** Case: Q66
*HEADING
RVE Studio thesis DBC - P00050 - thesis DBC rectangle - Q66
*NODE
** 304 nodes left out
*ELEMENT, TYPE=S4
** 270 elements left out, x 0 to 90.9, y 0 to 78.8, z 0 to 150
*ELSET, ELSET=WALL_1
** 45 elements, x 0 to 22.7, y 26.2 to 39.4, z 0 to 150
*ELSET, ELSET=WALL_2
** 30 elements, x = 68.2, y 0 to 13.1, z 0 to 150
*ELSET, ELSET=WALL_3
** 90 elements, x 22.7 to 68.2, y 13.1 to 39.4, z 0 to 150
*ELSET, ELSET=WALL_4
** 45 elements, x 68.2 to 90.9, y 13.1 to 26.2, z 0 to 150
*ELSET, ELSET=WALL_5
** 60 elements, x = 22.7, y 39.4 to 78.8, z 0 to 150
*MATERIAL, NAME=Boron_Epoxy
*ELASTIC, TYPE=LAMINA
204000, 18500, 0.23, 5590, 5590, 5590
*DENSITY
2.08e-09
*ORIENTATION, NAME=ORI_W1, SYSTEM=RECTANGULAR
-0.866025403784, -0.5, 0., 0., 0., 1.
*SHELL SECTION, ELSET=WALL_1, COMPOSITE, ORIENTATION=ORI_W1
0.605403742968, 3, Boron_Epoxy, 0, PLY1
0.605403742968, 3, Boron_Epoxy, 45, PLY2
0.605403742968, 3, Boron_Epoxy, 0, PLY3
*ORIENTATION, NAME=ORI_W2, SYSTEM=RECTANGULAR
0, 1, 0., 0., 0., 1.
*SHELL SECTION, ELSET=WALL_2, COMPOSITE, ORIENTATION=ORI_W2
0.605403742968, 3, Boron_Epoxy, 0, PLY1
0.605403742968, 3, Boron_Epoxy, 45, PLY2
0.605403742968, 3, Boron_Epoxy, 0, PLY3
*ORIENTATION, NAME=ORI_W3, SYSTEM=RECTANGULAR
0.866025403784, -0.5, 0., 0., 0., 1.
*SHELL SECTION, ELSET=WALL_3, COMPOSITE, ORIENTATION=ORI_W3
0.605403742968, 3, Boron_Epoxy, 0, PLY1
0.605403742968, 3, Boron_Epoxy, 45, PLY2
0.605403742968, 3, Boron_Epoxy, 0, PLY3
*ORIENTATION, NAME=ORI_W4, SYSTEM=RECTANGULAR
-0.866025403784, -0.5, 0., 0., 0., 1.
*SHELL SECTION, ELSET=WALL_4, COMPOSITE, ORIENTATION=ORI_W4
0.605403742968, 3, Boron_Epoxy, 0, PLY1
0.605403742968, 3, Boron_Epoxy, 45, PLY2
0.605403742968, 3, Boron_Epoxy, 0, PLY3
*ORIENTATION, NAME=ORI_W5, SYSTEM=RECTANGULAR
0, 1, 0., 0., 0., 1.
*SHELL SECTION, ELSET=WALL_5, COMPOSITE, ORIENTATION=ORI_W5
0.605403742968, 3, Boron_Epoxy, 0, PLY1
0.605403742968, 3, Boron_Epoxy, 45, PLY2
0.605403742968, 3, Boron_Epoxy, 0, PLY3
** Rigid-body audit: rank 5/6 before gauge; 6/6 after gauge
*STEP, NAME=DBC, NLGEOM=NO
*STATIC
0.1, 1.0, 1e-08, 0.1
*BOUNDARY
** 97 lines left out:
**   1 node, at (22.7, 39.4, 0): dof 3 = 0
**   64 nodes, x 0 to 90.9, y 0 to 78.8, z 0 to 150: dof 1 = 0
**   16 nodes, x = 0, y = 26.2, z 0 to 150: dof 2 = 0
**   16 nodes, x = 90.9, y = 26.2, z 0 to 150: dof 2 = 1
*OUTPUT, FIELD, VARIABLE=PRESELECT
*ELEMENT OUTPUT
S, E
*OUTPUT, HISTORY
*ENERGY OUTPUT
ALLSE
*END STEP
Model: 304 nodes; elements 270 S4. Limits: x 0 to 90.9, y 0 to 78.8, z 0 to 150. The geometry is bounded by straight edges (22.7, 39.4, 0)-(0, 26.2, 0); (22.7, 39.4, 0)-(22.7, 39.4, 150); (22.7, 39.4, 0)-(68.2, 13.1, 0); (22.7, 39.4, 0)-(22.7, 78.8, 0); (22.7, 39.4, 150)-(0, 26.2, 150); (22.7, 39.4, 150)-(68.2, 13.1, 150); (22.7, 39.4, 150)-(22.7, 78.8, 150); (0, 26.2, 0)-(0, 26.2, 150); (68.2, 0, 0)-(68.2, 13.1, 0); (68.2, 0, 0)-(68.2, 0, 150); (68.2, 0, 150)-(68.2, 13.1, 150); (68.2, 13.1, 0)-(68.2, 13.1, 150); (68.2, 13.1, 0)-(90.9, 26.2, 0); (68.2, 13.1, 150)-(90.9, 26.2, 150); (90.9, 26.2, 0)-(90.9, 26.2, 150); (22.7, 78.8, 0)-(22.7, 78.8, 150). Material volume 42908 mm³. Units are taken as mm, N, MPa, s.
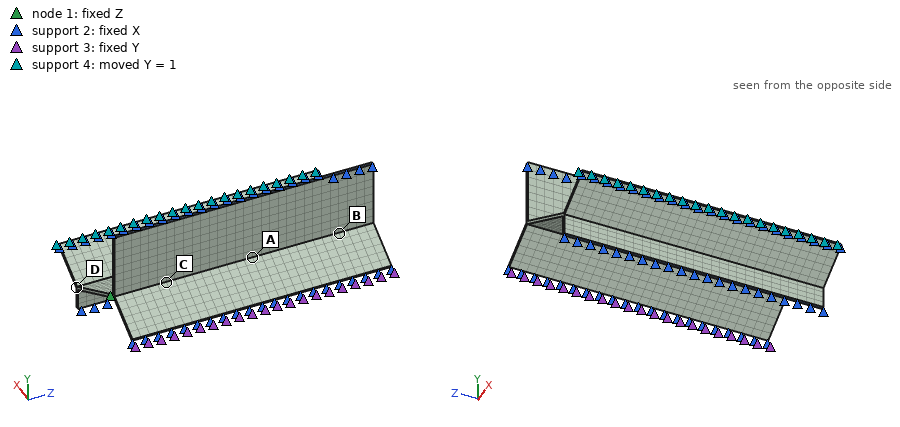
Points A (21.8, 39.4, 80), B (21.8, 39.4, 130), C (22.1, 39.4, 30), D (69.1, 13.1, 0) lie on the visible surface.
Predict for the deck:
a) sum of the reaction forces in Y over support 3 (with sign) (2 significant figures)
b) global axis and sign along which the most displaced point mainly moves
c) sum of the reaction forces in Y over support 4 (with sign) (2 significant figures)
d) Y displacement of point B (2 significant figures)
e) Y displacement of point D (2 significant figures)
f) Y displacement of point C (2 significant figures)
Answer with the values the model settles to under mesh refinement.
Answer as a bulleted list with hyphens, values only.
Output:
- -600 N
- +Y
- 600 N
- 0.40 mm
- 0.92 mm
- 0.41 mm
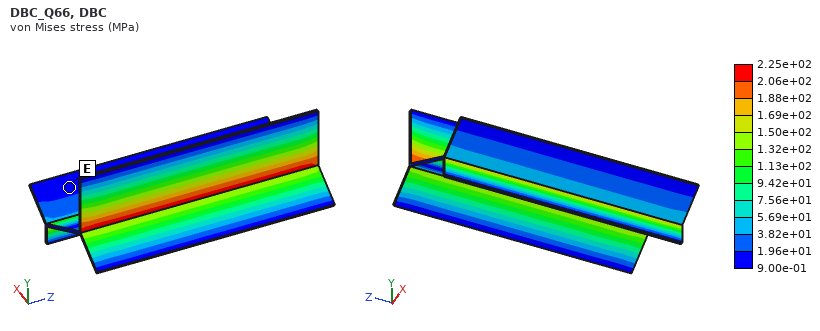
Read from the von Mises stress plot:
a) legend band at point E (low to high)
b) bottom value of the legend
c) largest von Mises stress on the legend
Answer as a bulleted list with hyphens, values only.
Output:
- 9.00e-01 to 1.96e+01 MPa
- 9.00e-01 MPa
- 2.25e+02 MPa
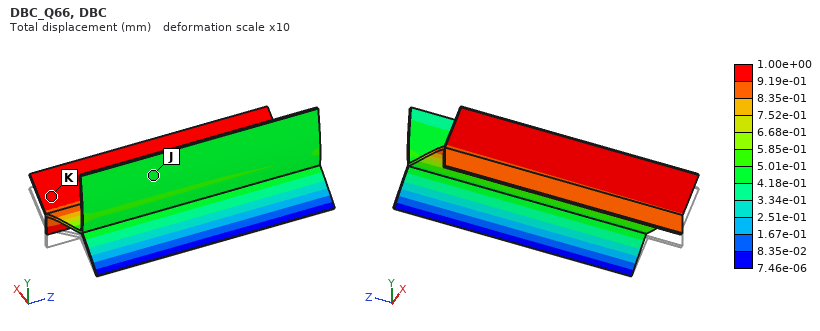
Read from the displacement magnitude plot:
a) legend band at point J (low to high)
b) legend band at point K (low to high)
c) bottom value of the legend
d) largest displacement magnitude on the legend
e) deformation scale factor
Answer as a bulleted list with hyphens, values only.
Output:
- 4.18e-01 to 5.01e-01 mm
- 9.19e-01 to 1.00e+00 mm
- 7.46e-06 mm
- 1.00e+00 mm
- 10
